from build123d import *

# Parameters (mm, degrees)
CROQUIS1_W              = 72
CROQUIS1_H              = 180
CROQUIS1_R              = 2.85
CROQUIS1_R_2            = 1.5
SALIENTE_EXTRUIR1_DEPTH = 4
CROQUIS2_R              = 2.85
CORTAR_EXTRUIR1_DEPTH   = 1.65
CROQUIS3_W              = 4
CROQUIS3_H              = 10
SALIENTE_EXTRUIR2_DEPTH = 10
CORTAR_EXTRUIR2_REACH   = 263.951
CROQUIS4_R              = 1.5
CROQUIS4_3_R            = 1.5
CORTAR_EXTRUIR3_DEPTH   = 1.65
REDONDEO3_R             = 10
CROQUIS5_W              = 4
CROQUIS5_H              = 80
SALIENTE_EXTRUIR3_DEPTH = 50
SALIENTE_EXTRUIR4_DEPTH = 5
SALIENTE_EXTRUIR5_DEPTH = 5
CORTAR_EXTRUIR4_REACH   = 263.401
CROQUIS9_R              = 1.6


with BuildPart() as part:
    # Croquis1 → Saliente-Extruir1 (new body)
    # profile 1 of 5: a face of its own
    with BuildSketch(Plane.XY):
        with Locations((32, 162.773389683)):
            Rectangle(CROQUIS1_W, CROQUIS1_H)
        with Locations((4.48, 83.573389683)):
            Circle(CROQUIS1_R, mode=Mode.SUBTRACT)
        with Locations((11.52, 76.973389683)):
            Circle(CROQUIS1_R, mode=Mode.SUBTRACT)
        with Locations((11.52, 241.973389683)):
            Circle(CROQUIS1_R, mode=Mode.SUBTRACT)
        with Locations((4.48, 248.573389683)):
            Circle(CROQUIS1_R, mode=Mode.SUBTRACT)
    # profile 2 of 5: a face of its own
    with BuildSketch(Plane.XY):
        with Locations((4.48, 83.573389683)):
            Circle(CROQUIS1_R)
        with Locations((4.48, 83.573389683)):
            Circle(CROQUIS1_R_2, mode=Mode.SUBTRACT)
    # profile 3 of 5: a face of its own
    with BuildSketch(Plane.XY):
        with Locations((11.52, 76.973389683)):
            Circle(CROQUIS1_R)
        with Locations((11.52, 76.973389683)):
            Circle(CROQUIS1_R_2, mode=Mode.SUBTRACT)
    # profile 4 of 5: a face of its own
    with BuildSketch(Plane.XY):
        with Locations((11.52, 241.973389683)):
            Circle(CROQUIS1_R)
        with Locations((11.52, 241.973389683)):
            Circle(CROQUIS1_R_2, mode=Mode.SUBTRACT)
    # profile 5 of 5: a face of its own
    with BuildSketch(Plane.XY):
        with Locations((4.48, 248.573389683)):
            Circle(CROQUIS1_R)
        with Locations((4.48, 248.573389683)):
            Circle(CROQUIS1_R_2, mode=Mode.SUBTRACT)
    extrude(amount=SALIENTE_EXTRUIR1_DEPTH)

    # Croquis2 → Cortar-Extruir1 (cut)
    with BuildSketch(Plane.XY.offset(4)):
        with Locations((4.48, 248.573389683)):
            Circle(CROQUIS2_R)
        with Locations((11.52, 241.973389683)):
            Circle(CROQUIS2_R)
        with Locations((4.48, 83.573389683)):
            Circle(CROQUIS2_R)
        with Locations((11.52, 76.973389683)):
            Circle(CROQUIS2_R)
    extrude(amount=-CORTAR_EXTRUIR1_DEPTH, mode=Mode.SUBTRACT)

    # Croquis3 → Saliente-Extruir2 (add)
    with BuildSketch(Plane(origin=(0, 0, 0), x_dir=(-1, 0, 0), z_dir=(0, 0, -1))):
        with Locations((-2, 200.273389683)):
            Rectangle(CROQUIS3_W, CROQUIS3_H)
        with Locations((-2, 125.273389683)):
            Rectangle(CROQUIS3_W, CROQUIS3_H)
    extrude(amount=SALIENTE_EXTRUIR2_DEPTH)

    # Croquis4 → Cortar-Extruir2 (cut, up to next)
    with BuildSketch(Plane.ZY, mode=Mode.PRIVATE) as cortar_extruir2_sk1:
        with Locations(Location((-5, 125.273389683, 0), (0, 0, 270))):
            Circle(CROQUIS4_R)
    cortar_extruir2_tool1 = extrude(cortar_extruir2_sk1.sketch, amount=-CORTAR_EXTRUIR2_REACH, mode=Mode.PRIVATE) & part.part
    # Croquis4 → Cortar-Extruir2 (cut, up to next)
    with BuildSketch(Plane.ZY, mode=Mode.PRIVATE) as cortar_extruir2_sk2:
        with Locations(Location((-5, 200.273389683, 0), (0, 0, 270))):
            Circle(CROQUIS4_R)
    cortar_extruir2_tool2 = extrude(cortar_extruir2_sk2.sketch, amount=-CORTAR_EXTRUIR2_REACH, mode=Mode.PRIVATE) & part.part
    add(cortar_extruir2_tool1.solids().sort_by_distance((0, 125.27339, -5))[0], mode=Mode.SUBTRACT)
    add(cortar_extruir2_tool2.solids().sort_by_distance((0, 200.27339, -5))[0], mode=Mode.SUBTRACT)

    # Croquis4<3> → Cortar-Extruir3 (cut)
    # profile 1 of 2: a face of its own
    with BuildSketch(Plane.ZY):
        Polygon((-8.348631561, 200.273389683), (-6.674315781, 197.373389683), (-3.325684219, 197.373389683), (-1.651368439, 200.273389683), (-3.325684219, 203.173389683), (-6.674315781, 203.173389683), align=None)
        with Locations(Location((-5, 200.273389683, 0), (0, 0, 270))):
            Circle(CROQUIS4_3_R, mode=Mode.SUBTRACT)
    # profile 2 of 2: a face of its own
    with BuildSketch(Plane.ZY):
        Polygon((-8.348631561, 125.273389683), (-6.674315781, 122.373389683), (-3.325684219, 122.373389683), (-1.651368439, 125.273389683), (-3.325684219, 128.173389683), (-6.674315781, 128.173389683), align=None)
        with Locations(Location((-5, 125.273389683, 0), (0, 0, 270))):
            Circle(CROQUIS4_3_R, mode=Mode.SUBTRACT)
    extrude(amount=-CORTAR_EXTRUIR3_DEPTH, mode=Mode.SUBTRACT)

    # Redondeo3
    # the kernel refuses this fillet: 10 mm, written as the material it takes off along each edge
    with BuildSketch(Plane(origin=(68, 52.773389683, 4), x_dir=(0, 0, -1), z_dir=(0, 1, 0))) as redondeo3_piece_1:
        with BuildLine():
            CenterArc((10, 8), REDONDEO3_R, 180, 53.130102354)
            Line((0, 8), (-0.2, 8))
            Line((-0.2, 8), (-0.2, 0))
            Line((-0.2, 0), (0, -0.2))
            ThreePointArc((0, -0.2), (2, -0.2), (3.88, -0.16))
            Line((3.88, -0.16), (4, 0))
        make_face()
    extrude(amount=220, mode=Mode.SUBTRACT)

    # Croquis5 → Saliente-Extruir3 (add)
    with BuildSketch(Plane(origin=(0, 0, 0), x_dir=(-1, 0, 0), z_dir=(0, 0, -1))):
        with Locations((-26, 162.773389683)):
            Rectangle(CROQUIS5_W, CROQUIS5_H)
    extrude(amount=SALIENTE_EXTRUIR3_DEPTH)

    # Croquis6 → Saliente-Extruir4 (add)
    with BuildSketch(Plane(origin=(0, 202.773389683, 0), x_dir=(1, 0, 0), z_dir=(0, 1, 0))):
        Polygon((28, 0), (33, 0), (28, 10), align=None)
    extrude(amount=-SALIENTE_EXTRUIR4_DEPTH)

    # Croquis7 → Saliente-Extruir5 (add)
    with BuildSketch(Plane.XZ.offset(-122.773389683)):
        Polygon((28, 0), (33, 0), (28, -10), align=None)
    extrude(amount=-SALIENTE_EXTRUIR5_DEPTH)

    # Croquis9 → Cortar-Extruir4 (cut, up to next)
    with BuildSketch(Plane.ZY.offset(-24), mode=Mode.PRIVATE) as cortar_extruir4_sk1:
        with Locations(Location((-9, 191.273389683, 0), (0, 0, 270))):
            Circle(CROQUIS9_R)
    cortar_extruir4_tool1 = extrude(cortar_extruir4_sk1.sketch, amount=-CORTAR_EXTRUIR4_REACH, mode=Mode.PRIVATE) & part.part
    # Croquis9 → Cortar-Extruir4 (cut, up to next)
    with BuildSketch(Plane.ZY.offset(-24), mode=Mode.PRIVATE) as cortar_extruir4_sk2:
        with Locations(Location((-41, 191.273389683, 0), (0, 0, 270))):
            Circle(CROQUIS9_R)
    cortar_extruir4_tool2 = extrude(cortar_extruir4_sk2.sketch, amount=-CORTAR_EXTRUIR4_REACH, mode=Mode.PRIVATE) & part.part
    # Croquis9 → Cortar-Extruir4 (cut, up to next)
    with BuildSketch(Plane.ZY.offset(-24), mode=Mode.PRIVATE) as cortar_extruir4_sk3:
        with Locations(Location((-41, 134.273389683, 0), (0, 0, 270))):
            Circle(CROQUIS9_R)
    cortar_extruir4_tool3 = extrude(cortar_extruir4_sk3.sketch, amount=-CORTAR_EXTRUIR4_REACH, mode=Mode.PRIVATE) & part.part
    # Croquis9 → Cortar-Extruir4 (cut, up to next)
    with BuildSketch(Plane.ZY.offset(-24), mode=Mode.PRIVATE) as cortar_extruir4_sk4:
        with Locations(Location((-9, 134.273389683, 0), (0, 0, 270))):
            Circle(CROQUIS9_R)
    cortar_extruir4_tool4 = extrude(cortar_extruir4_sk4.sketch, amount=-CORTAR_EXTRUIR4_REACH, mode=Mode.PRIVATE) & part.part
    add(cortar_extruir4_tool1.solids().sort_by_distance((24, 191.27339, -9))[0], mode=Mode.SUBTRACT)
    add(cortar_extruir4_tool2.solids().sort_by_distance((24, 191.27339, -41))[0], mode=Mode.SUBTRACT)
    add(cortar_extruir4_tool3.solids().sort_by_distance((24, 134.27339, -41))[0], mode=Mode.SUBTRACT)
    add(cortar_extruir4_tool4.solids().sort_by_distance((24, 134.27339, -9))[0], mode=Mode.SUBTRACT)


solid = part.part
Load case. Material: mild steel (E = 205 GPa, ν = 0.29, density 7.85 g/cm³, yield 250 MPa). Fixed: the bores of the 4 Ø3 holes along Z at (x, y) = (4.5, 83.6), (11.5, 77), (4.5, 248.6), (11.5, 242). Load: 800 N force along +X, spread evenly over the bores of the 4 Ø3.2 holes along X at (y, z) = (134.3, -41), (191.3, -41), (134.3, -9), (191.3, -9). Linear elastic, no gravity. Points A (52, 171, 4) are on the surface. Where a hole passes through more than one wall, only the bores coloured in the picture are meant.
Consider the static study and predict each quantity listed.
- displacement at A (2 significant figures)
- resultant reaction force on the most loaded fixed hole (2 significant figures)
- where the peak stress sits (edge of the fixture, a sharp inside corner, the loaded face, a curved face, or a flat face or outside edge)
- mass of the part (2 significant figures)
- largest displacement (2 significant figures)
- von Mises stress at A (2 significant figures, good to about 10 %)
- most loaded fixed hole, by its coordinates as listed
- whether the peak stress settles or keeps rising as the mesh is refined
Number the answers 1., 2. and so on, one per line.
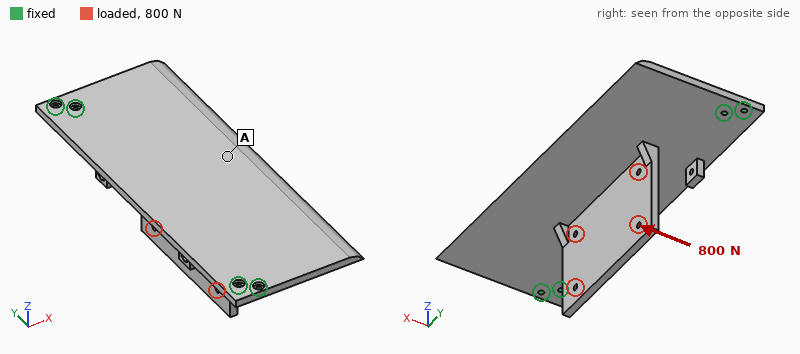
1. 0.29 mm
2. 1.0 kN
3. edge of the fixture
4. 520 g
5. 0.58 mm
6. 16 MPa
7. (11.5, 242)
8. keeps rising
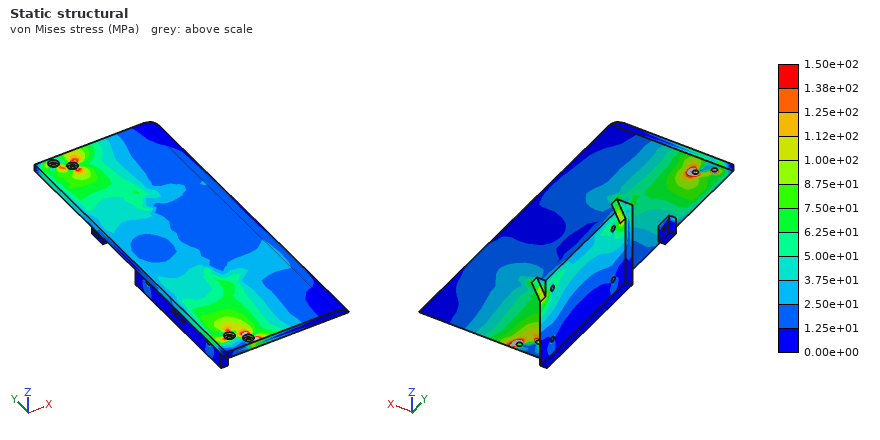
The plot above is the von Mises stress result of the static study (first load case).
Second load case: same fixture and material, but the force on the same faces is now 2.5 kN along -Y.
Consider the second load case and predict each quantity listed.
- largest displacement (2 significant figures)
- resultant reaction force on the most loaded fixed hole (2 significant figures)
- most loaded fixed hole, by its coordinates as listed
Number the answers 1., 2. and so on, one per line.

1. 0.18 mm
2. 1.2 kN
3. (11.5, 242)
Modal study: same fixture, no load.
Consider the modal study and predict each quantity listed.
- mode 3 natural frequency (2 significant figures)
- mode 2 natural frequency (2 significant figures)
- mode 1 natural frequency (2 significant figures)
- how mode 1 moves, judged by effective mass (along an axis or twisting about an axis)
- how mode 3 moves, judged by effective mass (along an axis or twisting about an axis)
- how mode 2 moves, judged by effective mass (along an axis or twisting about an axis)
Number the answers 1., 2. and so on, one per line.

1. 1000 Hz
2. 790 Hz
3. 420 Hz
4. along Z
5. twisting about X
6. along Z
